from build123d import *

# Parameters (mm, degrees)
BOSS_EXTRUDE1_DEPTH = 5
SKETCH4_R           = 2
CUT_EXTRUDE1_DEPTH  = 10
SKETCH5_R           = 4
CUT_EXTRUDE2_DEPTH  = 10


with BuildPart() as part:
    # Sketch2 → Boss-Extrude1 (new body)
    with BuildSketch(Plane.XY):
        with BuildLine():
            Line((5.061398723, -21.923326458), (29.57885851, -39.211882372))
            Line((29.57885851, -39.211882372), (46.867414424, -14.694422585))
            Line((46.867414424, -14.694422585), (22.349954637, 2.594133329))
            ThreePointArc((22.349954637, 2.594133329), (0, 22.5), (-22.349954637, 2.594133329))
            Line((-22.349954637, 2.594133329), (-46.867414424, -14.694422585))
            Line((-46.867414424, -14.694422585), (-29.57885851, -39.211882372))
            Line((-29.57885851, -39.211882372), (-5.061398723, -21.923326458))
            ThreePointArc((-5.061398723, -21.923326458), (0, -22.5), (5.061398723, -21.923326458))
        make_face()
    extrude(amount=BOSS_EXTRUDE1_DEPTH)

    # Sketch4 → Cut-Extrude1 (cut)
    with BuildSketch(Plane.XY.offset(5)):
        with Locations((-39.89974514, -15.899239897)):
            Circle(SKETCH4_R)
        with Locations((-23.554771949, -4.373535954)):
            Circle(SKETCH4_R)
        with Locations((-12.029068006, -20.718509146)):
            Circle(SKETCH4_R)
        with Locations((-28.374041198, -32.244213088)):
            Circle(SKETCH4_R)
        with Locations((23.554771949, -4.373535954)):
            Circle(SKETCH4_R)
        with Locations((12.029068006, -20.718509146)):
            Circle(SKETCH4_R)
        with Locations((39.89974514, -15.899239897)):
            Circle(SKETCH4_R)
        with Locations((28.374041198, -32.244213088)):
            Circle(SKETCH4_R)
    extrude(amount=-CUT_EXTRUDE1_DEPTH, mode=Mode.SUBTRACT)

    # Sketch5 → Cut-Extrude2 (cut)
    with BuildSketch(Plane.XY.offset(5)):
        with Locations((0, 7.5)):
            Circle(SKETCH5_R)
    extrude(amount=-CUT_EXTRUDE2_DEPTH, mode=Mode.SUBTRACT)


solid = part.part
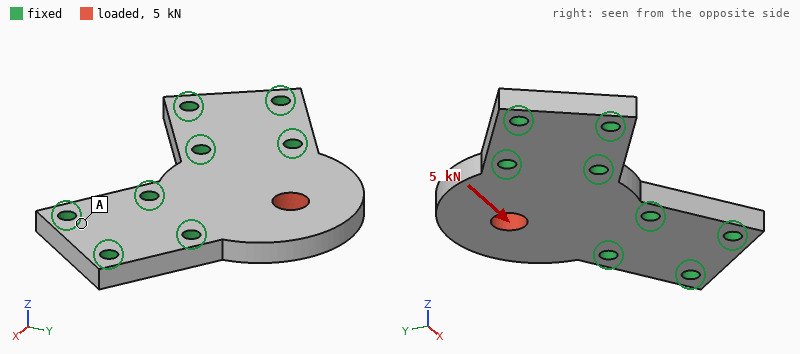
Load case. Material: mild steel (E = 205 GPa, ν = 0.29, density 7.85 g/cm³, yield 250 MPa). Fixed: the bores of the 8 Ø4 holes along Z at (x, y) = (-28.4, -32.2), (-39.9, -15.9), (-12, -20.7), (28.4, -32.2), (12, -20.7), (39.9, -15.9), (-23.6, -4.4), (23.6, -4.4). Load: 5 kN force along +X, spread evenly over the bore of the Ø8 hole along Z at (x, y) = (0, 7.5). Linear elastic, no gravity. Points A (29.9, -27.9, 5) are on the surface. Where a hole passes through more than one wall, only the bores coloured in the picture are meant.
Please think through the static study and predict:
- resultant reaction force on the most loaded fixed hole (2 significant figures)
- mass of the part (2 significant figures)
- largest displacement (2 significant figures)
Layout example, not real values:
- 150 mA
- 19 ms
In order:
- 2.2 kN
- 120 g
- 6.8 µm
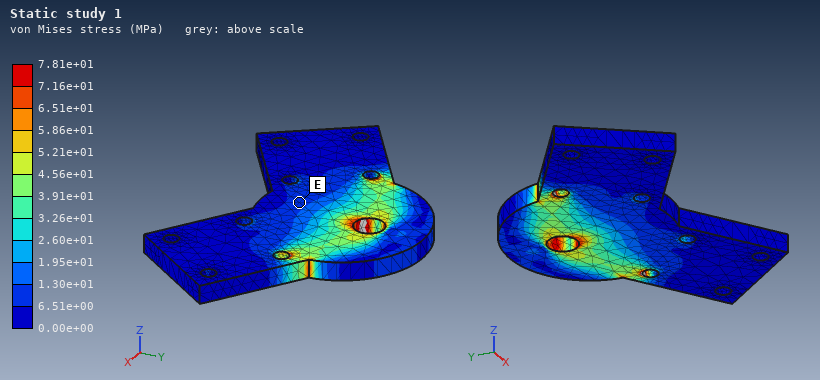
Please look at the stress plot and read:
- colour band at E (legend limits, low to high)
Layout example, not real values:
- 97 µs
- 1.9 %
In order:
- 6.51e+00 to 1.30e+01 MPa
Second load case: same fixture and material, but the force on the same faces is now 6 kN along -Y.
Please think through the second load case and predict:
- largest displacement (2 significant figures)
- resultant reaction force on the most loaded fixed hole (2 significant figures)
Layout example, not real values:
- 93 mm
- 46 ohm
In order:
- 6.3 µm
- 1.8 kN
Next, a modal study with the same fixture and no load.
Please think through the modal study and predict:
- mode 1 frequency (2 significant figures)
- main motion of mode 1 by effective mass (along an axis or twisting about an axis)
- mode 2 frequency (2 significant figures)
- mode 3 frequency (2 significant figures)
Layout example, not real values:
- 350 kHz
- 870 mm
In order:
- 5300 Hz
- along Z
- 14 kHz
- 18 kHz
